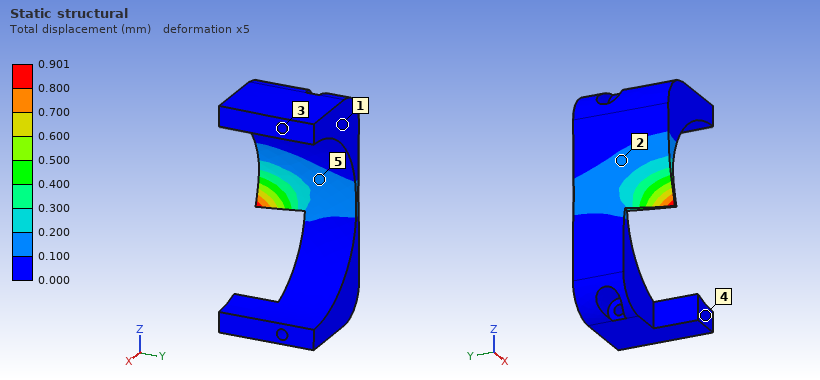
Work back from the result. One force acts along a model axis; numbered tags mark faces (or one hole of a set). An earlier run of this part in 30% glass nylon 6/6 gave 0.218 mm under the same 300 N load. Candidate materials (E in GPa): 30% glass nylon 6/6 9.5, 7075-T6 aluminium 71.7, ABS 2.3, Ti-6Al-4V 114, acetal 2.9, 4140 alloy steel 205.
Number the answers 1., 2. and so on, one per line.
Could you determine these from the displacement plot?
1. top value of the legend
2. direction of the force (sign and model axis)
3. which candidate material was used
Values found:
1. 0.901 mm
2. +X
3. ABS
